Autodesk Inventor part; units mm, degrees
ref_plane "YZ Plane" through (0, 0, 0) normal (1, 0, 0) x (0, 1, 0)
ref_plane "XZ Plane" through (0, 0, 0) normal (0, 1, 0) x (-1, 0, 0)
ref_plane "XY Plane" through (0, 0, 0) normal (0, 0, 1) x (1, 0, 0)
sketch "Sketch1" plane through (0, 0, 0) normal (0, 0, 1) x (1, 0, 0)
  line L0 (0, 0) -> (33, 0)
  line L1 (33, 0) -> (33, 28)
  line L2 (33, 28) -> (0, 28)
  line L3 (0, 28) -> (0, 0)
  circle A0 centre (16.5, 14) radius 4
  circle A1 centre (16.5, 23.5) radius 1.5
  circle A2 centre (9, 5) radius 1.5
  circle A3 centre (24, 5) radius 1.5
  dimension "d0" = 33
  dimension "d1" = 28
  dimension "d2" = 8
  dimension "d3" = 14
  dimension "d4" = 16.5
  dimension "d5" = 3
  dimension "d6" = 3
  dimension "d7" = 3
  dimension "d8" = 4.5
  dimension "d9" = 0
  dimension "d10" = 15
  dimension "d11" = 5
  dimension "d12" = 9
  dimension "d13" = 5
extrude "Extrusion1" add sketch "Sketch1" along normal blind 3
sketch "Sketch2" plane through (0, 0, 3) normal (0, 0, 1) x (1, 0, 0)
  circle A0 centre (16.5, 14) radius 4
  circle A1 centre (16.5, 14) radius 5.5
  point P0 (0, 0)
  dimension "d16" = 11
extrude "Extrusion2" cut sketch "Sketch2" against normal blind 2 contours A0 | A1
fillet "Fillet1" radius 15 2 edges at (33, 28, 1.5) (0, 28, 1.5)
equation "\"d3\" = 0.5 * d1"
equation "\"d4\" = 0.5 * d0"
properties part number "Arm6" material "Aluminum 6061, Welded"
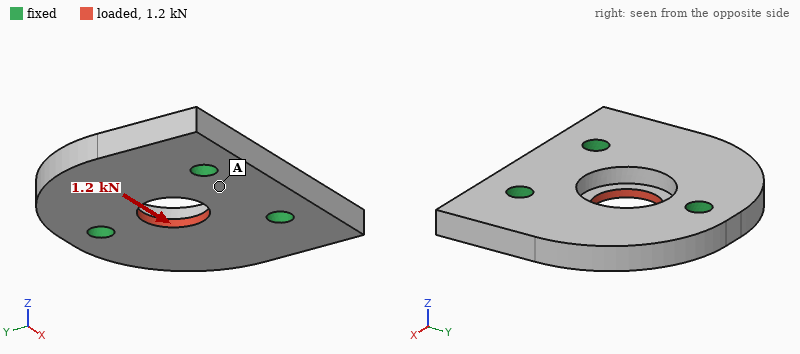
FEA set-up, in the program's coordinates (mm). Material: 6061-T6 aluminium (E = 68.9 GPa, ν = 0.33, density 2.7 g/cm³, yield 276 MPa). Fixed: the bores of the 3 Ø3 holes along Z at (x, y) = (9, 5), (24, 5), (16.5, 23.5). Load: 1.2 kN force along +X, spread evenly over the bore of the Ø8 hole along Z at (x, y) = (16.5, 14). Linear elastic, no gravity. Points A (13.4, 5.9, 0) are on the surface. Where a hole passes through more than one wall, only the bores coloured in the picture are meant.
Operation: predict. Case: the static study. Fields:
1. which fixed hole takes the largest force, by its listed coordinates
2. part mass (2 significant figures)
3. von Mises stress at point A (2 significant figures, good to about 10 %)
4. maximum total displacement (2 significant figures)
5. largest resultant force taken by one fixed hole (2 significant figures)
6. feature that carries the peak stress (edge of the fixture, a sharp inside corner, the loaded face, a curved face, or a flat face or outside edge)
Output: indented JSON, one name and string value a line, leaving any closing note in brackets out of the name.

{
  "which fixed hole takes the largest force, by its listed coordinates": "(16.5, 23.5)",
  "part mass": "5.9 g",
  "von Mises stress at point A": "12 MPa",
  "maximum total displacement": "6.6 µm",
  "largest resultant force taken by one fixed hole": "560 N",
  "feature that carries the peak stress": "the loaded face"
}
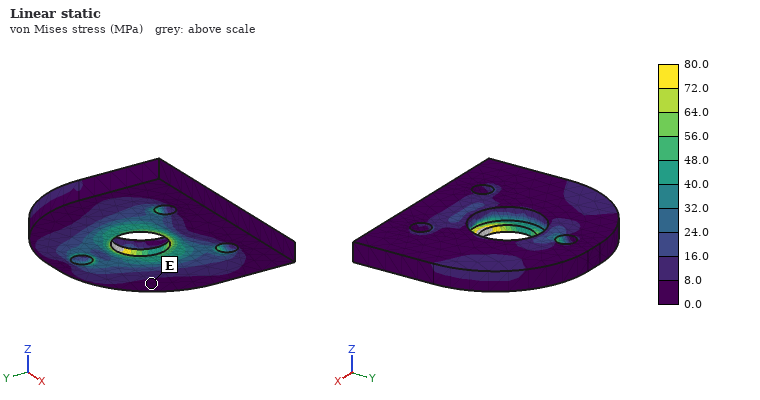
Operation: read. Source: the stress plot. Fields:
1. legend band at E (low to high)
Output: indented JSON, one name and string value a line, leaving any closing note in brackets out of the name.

{
  "legend band at E": "0.0 to 8.0 MPa"
}
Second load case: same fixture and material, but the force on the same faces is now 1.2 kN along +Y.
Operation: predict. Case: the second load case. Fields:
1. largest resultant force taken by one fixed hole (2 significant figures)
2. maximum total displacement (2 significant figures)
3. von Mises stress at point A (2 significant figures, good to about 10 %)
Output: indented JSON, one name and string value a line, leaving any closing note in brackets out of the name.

{
  "largest resultant force taken by one fixed hole": "430 N",
  "maximum total displacement": "5.9 µm",
  "von Mises stress at point A": "23 MPa"
}
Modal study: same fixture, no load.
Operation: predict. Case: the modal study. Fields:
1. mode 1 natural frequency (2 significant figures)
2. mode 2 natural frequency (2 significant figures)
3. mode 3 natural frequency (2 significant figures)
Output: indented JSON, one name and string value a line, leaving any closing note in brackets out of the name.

{
  "mode 1 natural frequency": "16 kHz",
  "mode 2 natural frequency": "17 kHz",
  "mode 3 natural frequency": "33 kHz"
}
